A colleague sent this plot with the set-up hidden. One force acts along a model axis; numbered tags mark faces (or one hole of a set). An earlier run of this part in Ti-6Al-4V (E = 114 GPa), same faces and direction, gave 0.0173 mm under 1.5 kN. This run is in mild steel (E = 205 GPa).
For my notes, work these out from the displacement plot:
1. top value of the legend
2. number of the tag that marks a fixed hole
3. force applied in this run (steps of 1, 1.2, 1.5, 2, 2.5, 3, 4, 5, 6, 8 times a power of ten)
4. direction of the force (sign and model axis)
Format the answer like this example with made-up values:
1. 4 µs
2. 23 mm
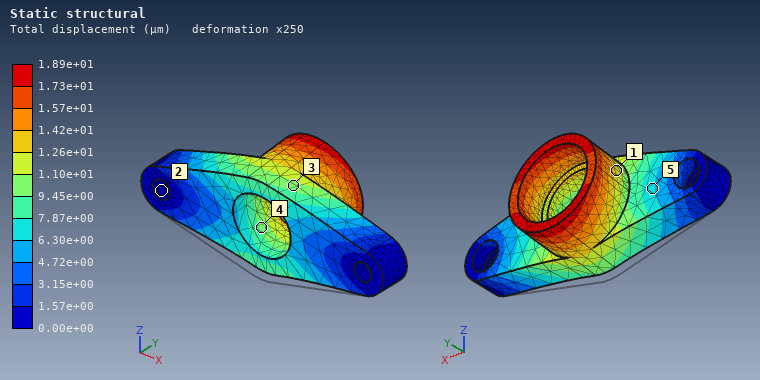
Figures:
1. 1.89e+01 µm
2. 2
3. 3 kN
4. +Z
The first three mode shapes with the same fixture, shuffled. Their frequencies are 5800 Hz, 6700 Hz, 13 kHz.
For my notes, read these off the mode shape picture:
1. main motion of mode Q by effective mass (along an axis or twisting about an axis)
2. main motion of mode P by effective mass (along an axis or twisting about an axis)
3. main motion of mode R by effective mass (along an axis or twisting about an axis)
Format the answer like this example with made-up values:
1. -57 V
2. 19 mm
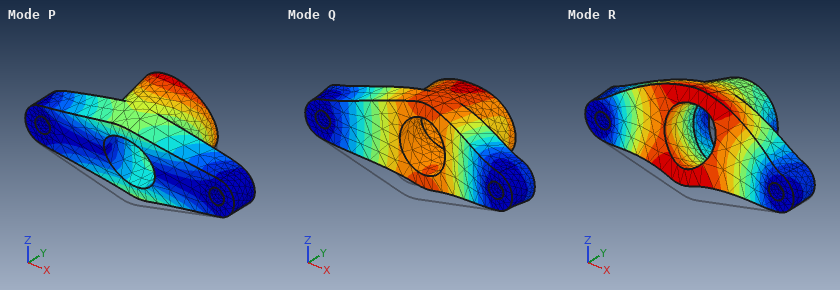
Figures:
1. along Y
2. along Z
3. along Z
